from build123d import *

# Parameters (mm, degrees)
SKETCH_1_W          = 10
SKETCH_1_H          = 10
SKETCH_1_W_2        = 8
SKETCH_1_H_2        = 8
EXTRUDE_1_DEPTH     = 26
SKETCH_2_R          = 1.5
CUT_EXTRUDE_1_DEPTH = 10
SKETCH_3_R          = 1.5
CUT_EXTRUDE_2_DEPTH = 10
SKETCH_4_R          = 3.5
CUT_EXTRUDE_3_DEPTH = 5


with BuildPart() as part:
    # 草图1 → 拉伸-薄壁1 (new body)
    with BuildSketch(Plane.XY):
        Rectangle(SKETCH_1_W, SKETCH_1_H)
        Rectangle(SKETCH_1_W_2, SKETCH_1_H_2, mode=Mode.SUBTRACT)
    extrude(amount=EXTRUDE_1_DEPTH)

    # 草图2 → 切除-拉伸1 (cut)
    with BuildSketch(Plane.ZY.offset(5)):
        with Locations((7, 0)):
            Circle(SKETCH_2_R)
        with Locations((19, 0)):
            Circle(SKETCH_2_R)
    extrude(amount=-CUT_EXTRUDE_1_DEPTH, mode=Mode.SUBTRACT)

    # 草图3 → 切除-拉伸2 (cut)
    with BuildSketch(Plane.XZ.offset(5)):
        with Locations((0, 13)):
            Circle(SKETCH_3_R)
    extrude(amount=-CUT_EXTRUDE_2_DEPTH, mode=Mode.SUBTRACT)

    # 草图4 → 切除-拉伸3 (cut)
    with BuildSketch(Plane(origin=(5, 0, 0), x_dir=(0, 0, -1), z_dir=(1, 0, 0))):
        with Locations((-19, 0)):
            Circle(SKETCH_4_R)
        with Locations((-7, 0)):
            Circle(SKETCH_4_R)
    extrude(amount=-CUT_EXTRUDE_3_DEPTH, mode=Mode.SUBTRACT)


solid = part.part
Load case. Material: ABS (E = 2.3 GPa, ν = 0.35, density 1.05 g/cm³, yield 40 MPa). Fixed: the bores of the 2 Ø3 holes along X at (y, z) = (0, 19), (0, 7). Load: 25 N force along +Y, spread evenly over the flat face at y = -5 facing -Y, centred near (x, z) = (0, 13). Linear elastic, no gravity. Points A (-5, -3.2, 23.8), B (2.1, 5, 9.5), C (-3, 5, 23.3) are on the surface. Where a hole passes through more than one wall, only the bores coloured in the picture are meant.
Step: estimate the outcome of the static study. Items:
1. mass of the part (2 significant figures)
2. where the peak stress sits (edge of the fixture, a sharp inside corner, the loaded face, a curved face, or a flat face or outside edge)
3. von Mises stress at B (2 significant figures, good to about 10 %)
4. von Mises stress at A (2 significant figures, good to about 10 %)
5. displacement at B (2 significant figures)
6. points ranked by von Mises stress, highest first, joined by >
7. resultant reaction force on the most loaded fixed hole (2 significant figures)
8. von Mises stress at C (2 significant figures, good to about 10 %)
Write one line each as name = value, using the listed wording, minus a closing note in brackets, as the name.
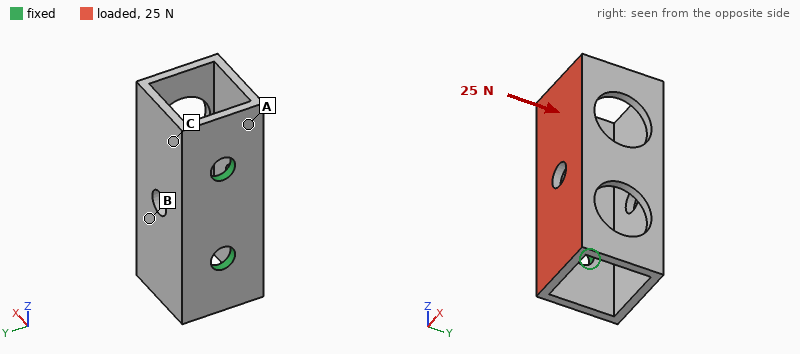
mass of the part = 0.87 g
where the peak stress sits = a flat face or outside edge
von Mises stress at B = 2.0 MPa
von Mises stress at A = 7.6 MPa
displacement at B = 0.25 mm
points ranked by von Mises stress, highest first, joined by > = A > C > B
resultant reaction force on the most loaded fixed hole = 13 N
von Mises stress at C = 4.5 MPa
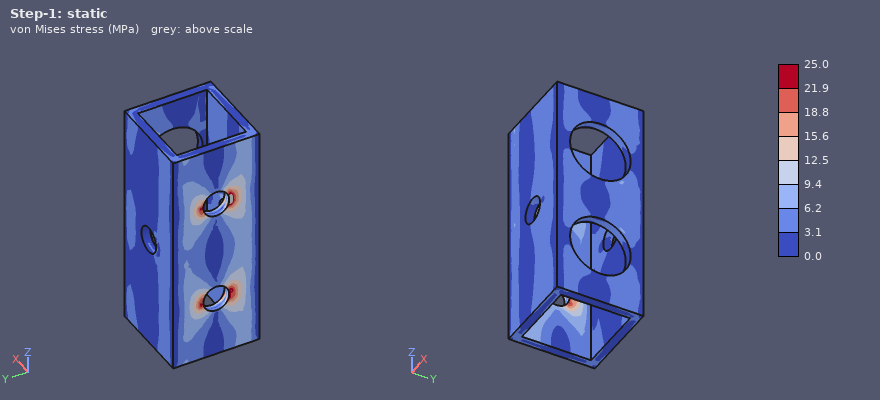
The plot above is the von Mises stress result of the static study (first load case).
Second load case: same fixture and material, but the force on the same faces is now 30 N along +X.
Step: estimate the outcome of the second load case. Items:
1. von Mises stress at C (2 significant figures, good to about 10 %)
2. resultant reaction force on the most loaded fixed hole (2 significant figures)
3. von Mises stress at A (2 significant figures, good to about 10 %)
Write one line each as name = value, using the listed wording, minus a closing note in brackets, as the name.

von Mises stress at C = 2.6 MPa
resultant reaction force on the most loaded fixed hole = 15 N
von Mises stress at A = 4.3 MPa
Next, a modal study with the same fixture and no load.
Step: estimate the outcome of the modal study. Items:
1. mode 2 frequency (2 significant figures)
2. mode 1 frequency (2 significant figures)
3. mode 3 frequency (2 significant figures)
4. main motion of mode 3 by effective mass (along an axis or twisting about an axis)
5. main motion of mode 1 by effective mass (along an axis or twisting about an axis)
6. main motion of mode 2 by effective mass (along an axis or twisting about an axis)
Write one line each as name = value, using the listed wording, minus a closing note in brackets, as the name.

mode 2 frequency = 3600 Hz
mode 1 frequency = 1600 Hz
mode 3 frequency = 4400 Hz
main motion of mode 3 by effective mass = twisting about X
main motion of mode 1 by effective mass = along Y
main motion of mode 2 by effective mass = along Z
